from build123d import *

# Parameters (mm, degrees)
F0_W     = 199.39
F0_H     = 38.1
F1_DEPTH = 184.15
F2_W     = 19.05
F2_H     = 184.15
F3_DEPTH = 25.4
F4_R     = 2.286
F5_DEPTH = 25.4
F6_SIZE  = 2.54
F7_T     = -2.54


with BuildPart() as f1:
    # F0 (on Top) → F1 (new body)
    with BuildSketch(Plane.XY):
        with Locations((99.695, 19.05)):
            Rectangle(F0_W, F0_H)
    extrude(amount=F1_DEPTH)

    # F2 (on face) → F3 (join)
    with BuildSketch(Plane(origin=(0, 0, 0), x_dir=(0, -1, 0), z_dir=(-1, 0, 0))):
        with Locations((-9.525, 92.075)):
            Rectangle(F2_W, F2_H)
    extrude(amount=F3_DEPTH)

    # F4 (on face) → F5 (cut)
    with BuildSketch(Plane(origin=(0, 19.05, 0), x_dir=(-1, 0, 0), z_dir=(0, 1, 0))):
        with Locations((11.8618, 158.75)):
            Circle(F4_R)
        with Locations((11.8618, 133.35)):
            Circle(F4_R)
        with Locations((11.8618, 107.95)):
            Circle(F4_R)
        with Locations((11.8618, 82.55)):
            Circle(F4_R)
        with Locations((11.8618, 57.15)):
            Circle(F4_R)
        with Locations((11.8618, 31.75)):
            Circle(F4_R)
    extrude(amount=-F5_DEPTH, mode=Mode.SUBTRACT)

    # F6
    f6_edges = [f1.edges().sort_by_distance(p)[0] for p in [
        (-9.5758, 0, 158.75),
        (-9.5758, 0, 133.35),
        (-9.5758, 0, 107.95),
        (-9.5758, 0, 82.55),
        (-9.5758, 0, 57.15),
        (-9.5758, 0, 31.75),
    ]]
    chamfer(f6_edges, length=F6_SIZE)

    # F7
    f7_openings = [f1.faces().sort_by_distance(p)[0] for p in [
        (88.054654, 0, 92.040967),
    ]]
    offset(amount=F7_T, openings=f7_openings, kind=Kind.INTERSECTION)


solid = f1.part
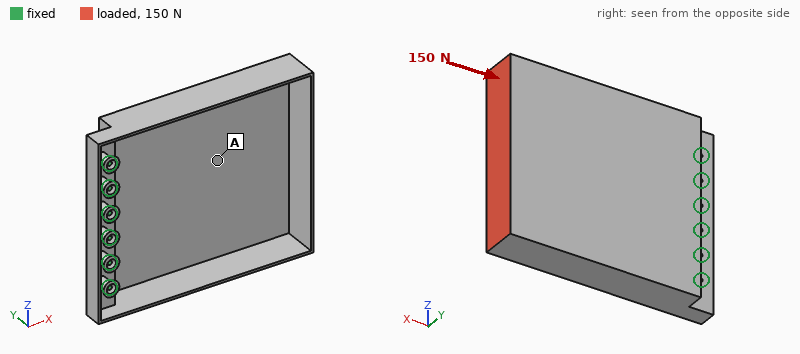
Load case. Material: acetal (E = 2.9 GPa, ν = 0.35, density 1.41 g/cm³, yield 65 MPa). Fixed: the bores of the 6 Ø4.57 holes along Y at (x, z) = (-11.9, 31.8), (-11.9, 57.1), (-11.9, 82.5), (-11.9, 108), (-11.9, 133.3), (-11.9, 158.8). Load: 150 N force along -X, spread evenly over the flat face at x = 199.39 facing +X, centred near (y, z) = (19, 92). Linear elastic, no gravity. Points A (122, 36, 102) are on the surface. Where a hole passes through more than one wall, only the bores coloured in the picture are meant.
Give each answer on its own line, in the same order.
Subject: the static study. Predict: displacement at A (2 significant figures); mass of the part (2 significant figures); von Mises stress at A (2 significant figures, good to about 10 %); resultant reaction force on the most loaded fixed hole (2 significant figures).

1.0 mm
260 g
1.3 MPa
110 N
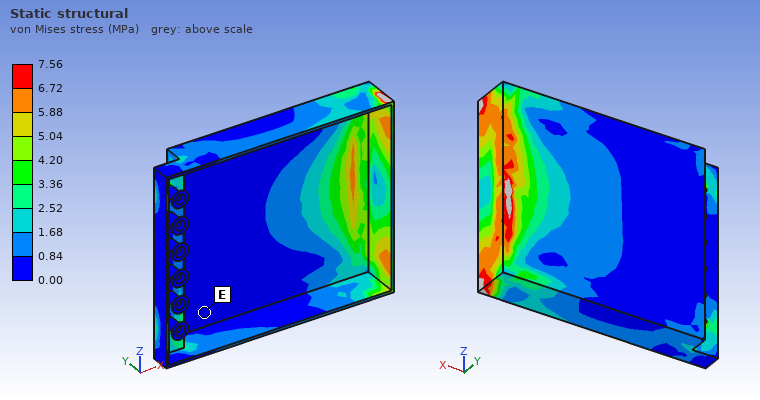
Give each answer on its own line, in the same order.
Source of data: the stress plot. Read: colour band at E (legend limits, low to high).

0.00 to 0.84 MPa
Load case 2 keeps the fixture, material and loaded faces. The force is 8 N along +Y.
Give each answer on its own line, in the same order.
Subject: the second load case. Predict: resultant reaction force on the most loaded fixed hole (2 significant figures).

67 N
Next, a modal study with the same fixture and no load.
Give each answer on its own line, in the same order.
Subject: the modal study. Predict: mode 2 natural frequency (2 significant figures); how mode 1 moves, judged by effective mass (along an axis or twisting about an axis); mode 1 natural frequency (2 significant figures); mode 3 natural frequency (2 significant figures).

37 Hz
along Y
27 Hz
150 Hz
